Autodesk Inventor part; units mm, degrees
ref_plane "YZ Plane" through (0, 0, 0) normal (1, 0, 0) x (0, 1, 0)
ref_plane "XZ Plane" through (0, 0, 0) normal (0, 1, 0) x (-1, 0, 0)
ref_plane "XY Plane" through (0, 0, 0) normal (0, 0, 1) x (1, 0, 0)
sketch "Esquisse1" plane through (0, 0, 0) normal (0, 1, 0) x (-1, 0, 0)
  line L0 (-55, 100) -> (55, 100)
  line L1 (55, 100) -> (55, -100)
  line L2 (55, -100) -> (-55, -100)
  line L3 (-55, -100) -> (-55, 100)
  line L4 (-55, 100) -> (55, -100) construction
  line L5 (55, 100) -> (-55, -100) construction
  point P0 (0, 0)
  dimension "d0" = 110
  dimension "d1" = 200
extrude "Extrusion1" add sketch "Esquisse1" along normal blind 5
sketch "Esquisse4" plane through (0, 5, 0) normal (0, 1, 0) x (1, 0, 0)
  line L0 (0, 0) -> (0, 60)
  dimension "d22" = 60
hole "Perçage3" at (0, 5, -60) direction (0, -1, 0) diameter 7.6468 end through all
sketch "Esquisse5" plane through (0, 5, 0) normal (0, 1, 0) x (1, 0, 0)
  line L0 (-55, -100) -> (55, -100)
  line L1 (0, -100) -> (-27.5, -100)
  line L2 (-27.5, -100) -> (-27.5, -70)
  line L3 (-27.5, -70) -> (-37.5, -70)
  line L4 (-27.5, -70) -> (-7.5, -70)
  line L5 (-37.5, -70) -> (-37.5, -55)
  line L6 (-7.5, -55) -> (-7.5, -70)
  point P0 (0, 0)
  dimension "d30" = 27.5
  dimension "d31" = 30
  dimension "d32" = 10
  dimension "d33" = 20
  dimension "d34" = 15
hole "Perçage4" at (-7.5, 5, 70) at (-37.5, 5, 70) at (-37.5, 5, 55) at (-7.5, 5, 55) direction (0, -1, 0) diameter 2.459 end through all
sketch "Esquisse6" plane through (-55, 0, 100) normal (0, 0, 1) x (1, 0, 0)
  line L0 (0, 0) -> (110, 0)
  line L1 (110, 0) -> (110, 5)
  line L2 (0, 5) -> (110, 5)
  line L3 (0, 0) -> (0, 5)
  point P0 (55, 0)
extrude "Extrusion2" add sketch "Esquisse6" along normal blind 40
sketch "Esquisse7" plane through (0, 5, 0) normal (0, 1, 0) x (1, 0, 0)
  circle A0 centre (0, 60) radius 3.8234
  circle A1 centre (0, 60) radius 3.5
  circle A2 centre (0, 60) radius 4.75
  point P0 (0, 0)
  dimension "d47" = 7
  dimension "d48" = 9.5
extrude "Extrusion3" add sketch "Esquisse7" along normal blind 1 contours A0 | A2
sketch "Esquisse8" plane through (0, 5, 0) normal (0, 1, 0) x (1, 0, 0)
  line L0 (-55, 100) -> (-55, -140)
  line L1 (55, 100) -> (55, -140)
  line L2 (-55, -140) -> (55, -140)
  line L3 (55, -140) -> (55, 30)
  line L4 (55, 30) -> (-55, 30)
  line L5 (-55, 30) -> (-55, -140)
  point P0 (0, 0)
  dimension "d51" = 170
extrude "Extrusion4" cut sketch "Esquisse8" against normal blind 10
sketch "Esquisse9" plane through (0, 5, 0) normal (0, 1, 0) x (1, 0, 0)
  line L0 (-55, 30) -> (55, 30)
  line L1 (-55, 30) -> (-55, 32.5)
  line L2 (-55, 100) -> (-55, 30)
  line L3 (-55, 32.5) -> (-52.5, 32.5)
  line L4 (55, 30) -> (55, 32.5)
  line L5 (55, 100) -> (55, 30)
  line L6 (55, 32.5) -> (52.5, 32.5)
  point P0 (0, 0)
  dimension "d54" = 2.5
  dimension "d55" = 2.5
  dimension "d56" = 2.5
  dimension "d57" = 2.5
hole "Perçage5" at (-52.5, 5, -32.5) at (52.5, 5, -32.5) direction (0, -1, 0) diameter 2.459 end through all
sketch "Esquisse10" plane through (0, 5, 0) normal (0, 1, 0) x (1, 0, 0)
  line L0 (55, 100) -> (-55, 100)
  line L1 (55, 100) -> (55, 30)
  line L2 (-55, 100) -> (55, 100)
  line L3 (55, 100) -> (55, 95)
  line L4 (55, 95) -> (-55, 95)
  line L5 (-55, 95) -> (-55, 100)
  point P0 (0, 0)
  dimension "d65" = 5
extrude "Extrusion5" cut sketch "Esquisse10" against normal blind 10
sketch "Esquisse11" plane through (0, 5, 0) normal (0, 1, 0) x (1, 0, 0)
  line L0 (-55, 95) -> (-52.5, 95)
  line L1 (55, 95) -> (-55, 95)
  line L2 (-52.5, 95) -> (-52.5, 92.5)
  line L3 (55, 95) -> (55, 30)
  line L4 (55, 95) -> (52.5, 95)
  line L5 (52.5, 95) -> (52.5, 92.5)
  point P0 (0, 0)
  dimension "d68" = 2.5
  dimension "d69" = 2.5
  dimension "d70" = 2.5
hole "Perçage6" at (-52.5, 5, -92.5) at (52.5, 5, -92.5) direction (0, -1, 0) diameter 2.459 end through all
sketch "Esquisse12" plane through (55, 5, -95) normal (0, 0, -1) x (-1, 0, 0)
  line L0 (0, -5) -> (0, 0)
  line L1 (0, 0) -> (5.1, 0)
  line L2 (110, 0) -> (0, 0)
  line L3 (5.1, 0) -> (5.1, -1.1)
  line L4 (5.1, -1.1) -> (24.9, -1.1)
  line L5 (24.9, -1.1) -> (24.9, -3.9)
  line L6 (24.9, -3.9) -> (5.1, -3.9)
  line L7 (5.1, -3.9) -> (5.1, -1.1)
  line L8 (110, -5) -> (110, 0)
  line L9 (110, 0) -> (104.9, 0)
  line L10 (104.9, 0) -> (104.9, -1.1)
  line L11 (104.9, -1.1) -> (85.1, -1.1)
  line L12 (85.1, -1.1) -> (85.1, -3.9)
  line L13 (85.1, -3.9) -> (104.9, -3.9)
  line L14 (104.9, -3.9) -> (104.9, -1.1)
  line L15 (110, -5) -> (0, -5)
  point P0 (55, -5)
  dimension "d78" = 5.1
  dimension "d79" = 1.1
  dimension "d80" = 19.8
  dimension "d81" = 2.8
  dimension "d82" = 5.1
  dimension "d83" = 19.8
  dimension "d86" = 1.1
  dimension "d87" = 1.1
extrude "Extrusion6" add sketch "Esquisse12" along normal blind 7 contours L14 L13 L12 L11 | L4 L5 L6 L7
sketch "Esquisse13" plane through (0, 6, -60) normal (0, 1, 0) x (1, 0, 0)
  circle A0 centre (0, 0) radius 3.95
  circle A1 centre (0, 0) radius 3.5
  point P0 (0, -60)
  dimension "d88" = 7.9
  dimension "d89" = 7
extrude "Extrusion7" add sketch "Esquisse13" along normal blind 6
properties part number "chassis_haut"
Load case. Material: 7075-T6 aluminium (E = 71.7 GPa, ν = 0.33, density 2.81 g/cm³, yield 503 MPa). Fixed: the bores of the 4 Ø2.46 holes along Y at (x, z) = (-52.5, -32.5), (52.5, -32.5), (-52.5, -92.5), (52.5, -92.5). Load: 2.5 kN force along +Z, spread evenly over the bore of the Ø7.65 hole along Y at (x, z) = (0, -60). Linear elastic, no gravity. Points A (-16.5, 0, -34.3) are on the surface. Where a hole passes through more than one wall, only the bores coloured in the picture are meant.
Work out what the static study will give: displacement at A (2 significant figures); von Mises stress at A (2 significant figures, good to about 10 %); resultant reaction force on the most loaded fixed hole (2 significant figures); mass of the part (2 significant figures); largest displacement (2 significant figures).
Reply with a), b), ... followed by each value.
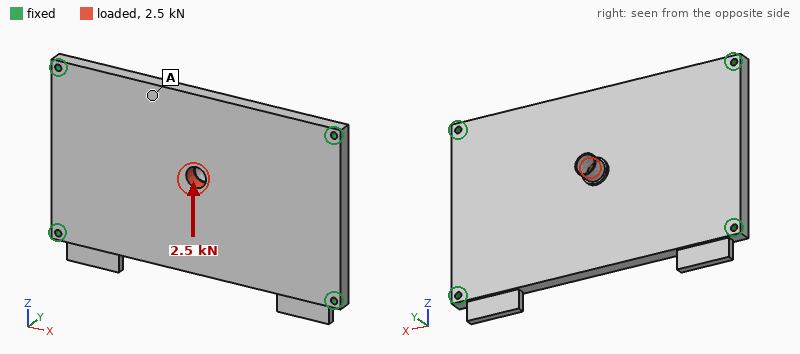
a) 9.4 µm
b) 5.2 MPa
c) 840 N
d) 100 g
e) 14 µm
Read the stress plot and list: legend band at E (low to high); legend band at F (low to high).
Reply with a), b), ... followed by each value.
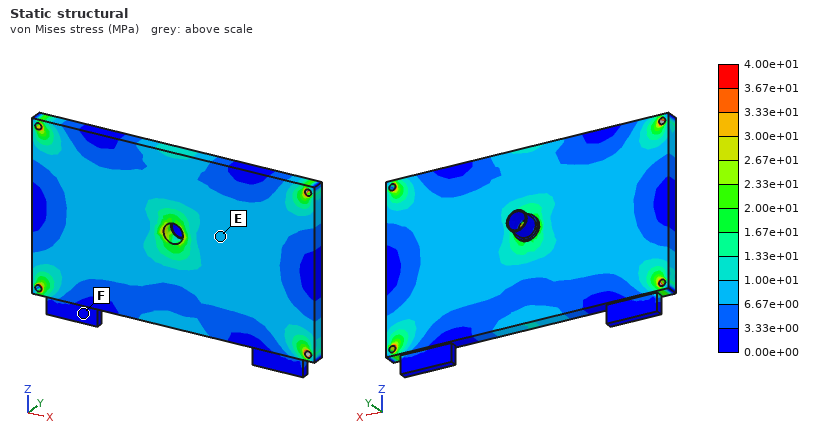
a) 6.67e+00 to 1.00e+01 MPa
b) 0.00e+00 to 3.33e+00 MPa
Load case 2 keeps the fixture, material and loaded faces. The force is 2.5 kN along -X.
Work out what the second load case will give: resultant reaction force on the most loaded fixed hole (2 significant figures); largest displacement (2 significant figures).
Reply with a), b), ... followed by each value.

a) 680 N
b) 8.2 µm
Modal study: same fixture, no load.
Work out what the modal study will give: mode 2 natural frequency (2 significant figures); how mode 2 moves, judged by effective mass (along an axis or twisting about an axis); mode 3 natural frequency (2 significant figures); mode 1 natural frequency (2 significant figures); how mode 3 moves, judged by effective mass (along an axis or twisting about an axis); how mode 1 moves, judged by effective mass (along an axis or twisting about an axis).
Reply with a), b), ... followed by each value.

a) 3100 Hz
b) twisting about X
c) 4600 Hz
d) 1700 Hz
e) twisting about Z
f) along Y
